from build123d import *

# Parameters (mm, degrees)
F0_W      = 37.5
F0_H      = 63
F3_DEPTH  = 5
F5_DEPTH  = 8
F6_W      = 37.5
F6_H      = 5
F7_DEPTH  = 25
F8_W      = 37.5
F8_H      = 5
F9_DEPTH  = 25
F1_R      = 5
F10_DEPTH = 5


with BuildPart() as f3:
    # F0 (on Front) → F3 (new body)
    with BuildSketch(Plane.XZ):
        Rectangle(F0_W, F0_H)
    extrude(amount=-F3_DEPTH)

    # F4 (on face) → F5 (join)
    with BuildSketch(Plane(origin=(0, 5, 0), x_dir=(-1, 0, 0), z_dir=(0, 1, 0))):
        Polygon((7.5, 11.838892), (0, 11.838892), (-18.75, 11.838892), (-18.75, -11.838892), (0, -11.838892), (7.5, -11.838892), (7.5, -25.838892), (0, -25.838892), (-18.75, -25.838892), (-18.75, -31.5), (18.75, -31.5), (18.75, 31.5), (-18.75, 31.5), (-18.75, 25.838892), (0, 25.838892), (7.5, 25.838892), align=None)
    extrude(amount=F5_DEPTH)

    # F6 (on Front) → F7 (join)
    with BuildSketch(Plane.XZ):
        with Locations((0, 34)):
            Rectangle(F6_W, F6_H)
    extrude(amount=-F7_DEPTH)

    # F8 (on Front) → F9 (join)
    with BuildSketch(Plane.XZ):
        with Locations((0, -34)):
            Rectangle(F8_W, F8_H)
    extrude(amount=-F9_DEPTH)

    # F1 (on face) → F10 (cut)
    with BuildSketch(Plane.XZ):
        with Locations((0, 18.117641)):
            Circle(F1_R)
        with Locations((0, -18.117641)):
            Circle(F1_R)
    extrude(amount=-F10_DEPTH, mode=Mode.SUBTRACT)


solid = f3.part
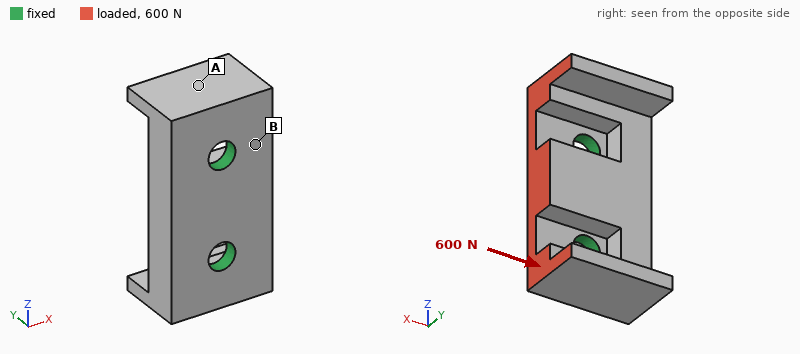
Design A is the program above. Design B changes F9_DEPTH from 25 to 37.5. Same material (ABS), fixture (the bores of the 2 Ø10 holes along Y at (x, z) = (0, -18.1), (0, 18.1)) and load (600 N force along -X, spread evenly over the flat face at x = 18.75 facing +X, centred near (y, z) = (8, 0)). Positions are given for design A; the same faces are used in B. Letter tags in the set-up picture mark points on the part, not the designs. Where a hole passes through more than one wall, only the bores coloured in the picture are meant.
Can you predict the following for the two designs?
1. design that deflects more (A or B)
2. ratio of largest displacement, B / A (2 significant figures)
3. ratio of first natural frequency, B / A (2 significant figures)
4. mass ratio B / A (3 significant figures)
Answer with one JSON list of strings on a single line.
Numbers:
["B", "2.4", "0.57", "1.07"]
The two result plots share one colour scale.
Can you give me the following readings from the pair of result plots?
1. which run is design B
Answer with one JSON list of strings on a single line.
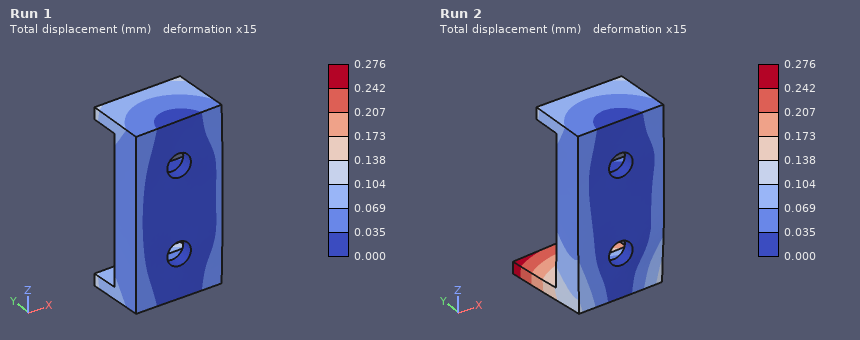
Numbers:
["Run 2"]
